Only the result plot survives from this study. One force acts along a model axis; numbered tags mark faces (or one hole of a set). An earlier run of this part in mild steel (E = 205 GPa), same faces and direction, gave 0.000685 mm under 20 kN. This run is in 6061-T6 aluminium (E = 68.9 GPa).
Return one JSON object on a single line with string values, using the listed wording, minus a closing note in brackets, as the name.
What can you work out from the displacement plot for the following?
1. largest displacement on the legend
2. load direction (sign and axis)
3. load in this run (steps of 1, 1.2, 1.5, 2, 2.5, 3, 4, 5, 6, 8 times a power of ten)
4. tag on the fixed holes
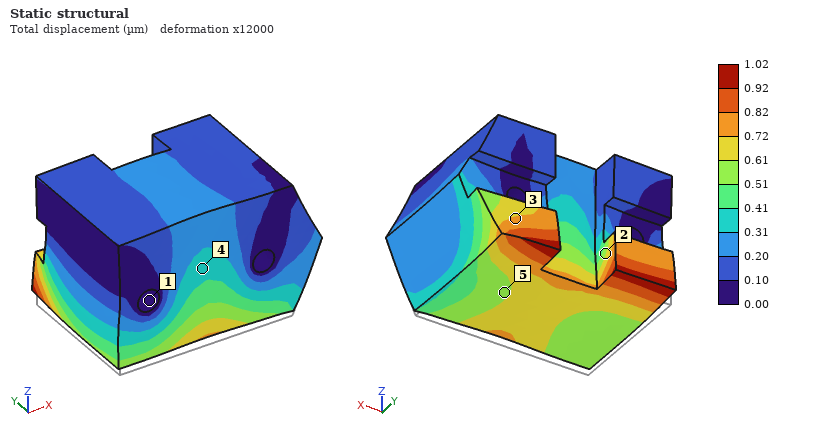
{"largest displacement on the legend": "1.02 µm", "load direction": "+Z", "load in this run": "10 kN", "tag on the fixed holes": "1"}
